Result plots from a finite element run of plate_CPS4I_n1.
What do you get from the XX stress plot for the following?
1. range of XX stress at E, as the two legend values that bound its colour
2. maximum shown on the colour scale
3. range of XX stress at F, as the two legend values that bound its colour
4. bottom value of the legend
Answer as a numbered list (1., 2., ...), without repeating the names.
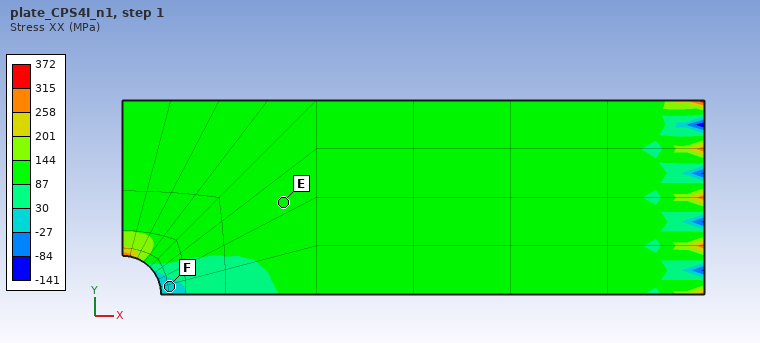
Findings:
1. 87 to 144 MPa
2. 372 MPa
3. -27 to 30 MPa
4. -141 MPa
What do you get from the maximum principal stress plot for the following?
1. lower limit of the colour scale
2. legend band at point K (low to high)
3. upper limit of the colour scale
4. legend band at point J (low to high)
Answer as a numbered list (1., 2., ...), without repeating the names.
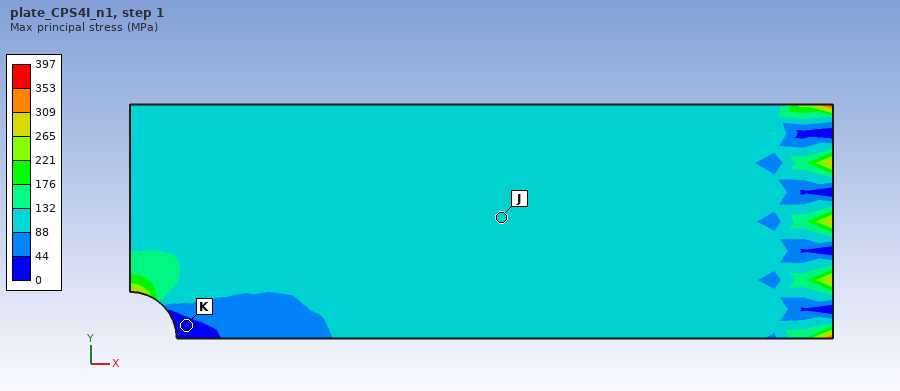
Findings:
1. 0 MPa
2. 0 to 44 MPa
3. 397 MPa
4. 88 to 132 MPa
